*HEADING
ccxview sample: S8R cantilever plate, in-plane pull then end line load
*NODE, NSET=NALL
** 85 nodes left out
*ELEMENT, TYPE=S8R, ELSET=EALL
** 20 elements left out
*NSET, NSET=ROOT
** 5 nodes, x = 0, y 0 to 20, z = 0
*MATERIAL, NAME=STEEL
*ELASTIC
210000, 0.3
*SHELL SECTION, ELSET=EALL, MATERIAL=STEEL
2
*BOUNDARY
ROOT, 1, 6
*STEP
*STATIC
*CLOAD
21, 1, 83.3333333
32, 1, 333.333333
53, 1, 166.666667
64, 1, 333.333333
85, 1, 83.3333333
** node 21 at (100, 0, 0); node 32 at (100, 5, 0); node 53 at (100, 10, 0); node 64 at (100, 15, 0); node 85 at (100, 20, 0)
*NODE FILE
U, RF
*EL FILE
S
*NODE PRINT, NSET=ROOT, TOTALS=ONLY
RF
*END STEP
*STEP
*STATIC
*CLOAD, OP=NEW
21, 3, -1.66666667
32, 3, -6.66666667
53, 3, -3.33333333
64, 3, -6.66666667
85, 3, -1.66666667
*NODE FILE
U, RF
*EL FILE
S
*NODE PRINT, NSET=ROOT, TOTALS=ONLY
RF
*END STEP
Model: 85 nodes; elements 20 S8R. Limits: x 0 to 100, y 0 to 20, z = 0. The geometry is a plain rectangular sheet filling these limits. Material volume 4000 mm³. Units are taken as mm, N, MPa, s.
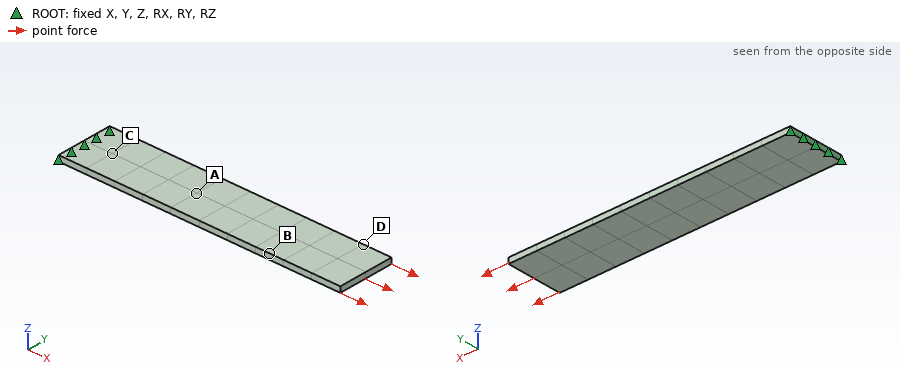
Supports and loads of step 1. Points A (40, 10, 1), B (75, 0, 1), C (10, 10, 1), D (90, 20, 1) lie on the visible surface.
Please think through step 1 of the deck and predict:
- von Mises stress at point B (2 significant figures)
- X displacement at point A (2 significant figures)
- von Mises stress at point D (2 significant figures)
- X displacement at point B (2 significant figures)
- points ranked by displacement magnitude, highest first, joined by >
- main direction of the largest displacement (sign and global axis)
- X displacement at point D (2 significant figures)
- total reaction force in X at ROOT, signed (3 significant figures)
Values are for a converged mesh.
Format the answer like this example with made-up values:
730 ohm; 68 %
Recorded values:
25 MPa; 0.0047 mm; 26 MPa; 0.0089 mm; D > B > A > C; +X; 0.011 mm; -1000 N
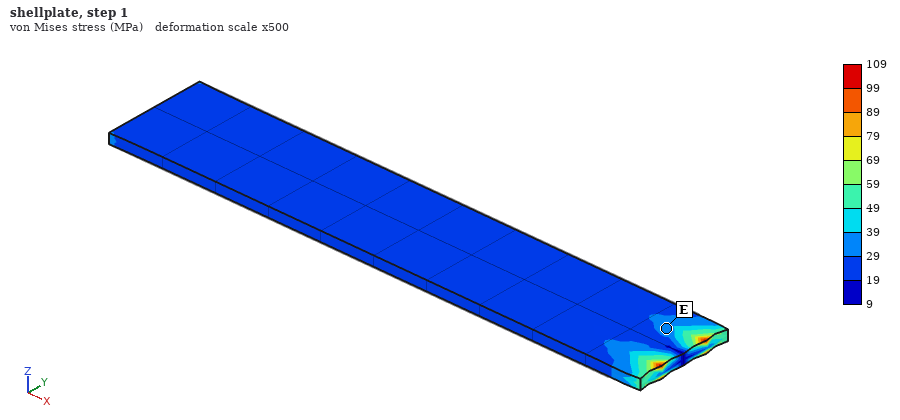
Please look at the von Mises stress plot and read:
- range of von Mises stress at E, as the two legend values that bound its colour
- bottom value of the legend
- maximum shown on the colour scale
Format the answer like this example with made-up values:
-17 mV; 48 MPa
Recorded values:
29 to 39 MPa; 9 MPa; 109 MPa
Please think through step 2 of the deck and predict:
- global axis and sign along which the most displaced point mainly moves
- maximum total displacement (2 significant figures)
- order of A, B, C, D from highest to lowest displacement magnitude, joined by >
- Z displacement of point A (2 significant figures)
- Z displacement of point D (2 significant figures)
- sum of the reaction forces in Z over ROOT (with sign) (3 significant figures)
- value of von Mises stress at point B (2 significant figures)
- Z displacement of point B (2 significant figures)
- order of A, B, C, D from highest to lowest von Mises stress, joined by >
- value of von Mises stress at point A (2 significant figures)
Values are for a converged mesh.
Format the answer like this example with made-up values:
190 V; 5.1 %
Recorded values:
-Z; 2.3 mm; D > B > A > C; -0.48 mm; -2.0 mm; 20.0 N; 38 MPa; -1.5 mm; C > A > B > D; 90 MPa
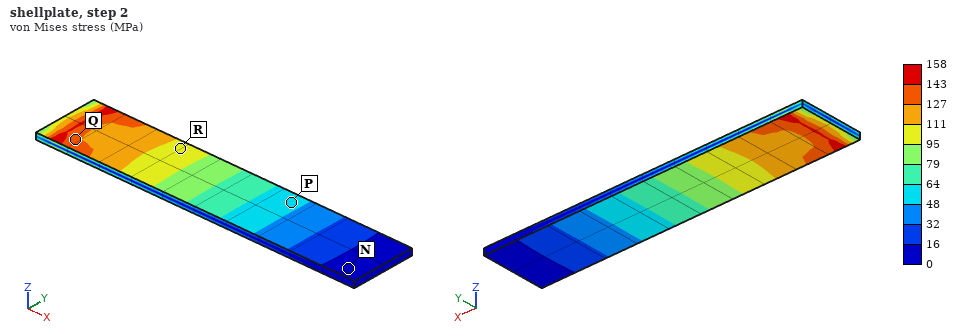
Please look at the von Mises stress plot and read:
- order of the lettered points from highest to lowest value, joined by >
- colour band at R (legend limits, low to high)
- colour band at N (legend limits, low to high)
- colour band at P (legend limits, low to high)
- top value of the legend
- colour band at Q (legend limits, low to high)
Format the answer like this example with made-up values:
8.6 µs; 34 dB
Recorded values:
Q > R > P > N; 95 to 111 MPa; 0 to 16 MPa; 48 to 64 MPa; 158 MPa; 127 to 143 MPa
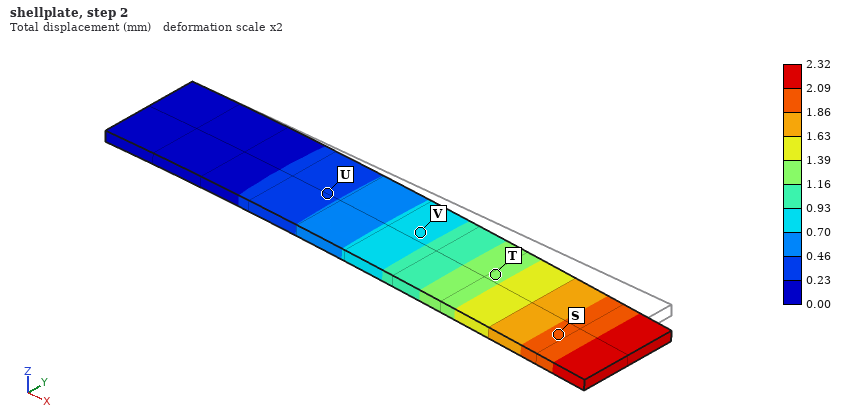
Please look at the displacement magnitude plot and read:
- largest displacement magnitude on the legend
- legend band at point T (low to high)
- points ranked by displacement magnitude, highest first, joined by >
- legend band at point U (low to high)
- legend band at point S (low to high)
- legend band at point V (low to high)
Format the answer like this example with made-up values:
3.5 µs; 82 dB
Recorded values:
2.32 mm; 1.16 to 1.39 mm; S > T > V > U; 0.23 to 0.46 mm; 1.86 to 2.09 mm; 0.70 to 0.93 mm
